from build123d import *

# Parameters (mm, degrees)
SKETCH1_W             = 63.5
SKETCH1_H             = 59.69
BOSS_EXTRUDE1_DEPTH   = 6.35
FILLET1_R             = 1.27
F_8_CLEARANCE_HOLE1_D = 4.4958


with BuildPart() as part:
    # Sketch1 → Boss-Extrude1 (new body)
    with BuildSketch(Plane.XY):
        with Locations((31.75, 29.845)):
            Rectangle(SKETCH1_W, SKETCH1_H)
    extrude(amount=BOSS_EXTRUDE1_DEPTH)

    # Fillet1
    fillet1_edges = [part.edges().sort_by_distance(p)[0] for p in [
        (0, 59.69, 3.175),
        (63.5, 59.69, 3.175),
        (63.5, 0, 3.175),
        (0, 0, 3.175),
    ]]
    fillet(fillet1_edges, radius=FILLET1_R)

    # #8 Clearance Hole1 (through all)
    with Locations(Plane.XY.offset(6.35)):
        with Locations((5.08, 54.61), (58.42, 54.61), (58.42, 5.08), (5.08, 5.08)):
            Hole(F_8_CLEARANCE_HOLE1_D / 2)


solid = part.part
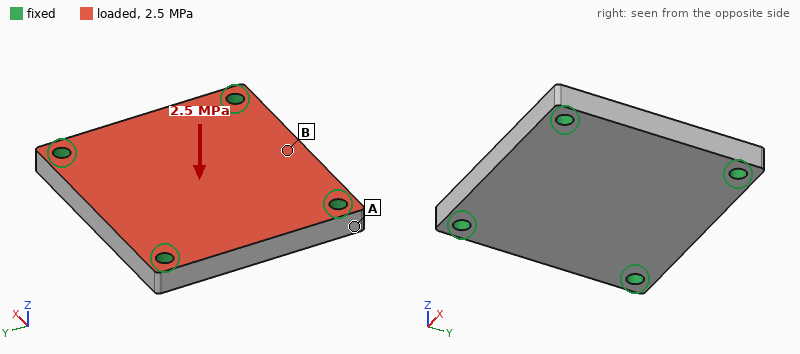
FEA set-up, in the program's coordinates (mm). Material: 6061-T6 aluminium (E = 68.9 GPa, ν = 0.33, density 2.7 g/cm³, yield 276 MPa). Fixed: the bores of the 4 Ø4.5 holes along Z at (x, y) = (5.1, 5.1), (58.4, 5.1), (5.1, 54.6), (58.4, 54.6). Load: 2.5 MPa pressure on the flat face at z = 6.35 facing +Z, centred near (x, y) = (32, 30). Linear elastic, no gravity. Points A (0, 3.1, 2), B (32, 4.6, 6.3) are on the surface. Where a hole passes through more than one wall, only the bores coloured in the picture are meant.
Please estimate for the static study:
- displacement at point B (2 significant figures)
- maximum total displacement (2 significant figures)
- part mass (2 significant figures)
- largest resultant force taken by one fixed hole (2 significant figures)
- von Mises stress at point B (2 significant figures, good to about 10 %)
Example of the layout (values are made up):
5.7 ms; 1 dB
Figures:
56 µm; 89 µm; 64 g; 2.3 kN; 56 MPa
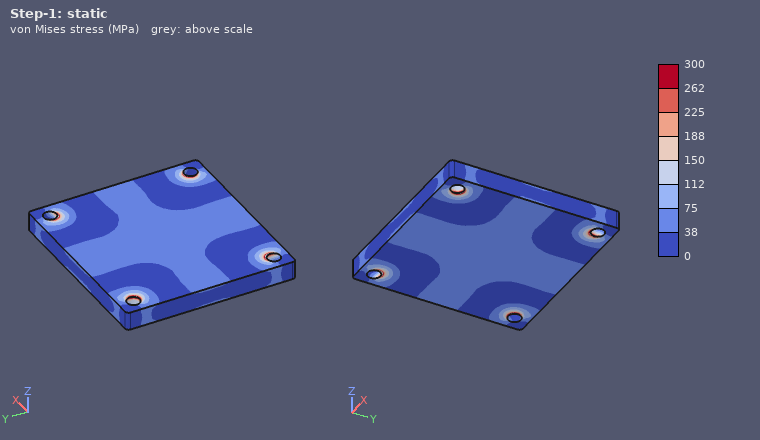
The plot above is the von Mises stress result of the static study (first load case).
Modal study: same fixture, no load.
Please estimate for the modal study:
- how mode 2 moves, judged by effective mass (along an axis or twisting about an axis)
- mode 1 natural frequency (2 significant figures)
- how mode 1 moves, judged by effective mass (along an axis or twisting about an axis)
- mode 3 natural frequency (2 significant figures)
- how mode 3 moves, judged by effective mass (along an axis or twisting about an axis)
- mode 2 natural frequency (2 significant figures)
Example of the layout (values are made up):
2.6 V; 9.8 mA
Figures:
twisting about X; 7700 Hz; along Z; 13 kHz; twisting about Y; 12 kHz
